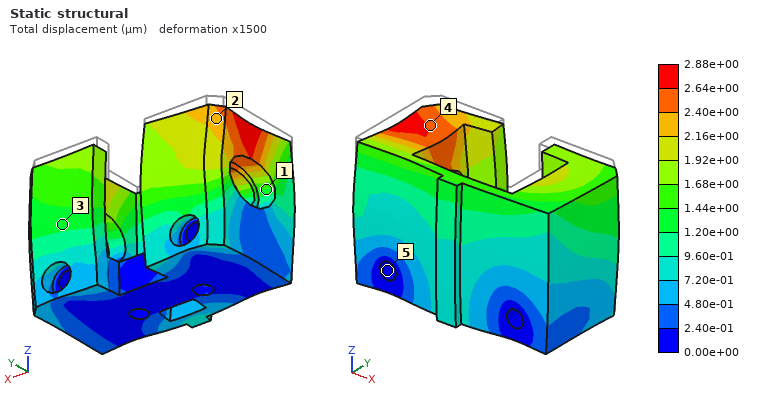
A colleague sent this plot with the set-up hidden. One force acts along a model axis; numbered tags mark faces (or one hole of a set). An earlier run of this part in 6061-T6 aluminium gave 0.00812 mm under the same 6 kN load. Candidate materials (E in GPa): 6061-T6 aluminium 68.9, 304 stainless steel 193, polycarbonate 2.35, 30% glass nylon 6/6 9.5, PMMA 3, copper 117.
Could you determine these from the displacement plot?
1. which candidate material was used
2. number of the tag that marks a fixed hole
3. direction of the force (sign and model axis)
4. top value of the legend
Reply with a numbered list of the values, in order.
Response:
1. 304 stainless steel
2. 5
3. -Z
4. 2.88e+00 µm
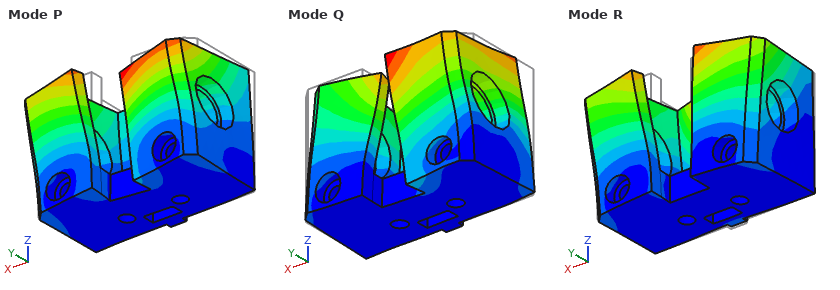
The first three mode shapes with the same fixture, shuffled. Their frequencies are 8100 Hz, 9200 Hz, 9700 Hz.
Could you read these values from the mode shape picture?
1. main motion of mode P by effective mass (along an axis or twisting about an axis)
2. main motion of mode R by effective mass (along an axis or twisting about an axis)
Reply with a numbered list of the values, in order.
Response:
1. along X
2. along Y
